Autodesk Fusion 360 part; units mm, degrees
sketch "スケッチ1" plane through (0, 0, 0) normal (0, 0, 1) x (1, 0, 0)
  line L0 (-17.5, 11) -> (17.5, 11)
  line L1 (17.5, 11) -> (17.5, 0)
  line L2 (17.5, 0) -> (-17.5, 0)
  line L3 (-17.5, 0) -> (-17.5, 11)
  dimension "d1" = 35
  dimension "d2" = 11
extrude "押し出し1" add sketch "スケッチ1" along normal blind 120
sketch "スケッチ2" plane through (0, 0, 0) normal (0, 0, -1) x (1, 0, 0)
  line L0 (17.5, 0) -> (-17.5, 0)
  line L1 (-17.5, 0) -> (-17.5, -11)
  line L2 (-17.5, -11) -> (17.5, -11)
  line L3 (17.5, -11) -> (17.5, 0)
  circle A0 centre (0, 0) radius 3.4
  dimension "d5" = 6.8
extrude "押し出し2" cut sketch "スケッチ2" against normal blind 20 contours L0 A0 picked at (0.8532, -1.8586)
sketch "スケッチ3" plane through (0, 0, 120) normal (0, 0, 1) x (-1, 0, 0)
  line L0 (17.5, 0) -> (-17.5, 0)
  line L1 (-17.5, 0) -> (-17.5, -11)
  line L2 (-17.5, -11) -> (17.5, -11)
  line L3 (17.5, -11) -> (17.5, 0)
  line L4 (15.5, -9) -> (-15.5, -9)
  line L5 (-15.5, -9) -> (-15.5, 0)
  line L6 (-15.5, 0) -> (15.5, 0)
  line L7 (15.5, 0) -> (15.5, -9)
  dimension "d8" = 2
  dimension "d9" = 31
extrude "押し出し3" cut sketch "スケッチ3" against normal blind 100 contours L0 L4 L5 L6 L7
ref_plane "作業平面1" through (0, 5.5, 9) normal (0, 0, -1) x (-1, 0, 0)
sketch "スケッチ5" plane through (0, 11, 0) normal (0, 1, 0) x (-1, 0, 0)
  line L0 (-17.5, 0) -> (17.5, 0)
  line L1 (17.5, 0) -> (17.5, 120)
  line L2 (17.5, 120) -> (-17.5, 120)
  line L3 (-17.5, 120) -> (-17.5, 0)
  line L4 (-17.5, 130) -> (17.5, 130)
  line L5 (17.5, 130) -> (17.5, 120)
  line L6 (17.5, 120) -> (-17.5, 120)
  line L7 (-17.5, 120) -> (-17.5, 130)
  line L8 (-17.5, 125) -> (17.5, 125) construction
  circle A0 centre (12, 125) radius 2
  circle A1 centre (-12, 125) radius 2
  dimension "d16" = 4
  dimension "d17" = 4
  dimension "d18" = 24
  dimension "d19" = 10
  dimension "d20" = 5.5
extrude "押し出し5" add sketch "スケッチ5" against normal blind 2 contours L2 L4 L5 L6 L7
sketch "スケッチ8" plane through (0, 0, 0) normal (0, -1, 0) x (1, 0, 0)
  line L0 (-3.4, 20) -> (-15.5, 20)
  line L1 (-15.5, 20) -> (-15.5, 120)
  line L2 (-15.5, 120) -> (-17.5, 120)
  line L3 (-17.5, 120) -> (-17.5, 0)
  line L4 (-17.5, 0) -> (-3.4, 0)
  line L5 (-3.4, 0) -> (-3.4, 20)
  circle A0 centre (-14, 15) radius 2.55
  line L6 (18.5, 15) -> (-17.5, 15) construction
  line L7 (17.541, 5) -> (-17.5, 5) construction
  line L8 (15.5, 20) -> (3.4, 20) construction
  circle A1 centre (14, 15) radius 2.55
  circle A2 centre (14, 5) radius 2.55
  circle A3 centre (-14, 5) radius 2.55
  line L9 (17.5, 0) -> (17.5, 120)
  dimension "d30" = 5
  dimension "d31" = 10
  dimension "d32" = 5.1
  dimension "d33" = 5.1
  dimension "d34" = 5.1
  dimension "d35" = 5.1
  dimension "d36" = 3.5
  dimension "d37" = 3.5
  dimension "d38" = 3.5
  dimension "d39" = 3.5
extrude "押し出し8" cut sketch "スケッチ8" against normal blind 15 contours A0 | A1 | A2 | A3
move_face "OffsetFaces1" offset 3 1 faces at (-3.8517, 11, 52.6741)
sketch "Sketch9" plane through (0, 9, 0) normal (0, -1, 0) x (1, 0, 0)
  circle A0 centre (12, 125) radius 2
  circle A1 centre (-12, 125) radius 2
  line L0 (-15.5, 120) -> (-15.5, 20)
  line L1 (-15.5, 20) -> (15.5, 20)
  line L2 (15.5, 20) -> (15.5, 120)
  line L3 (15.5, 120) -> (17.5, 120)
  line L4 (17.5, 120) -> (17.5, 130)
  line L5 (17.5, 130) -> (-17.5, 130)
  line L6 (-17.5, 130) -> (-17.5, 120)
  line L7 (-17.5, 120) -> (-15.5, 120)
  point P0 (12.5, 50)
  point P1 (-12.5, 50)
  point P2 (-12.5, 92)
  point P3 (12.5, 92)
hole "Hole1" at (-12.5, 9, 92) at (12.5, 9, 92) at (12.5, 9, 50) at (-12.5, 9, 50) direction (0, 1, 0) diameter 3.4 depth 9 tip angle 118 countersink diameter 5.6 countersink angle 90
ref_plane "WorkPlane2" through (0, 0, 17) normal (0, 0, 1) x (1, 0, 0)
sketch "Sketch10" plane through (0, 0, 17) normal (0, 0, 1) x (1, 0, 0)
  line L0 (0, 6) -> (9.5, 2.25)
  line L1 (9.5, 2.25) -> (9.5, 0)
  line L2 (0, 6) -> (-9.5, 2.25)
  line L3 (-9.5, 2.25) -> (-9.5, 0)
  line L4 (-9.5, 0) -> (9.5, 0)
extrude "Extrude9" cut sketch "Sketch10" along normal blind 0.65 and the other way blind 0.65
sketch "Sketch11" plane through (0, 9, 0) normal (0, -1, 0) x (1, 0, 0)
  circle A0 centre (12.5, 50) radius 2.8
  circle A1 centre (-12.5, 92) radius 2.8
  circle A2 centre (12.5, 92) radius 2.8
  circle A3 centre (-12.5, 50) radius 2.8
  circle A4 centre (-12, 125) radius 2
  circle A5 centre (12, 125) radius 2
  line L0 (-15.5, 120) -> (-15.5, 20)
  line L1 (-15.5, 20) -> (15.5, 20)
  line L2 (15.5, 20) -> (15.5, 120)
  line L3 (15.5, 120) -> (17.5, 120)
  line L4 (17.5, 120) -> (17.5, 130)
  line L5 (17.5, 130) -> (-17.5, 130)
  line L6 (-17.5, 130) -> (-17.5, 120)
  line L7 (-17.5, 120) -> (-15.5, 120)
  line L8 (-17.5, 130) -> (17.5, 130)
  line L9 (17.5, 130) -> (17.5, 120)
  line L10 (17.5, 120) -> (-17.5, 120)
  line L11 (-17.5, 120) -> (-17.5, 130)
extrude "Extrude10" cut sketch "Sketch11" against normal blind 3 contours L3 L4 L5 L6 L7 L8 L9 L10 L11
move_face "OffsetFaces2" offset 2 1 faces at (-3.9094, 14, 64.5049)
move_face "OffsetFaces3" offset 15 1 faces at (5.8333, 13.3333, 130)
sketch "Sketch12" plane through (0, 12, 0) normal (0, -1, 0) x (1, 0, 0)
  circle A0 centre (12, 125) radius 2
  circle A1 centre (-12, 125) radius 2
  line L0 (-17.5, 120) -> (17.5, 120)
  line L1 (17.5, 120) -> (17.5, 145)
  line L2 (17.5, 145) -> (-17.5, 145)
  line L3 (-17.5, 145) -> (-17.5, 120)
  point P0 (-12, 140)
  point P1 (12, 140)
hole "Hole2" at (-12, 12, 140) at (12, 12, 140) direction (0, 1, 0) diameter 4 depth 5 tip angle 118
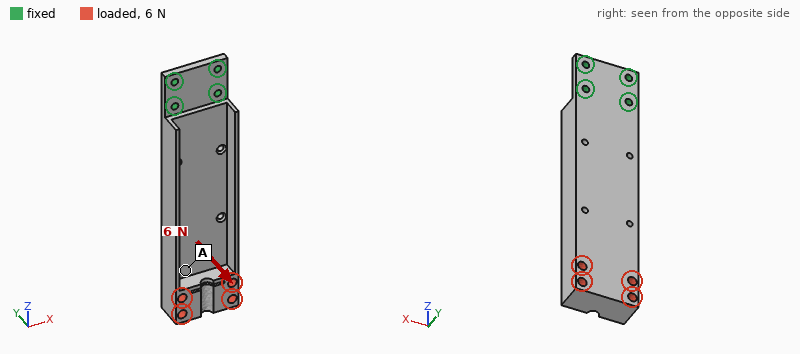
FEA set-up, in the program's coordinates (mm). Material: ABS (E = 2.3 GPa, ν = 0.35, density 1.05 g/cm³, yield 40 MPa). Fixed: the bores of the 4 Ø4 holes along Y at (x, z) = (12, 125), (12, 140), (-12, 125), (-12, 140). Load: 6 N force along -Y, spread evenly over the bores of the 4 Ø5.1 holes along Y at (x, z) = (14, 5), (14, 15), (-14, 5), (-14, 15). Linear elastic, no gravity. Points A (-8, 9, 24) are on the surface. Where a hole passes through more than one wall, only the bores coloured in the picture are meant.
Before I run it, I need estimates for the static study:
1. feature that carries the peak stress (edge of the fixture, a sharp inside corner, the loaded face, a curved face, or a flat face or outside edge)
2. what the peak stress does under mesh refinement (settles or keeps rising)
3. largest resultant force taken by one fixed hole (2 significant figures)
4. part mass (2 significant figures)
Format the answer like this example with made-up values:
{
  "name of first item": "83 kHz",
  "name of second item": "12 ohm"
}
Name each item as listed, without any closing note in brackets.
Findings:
{
  "feature that carries the peak stress": "edge of the fixture",
  "what the peak stress does under mesh refinement": "keeps rising",
  "largest resultant force taken by one fixed hole": "11 N",
  "part mass": "43 g"
}
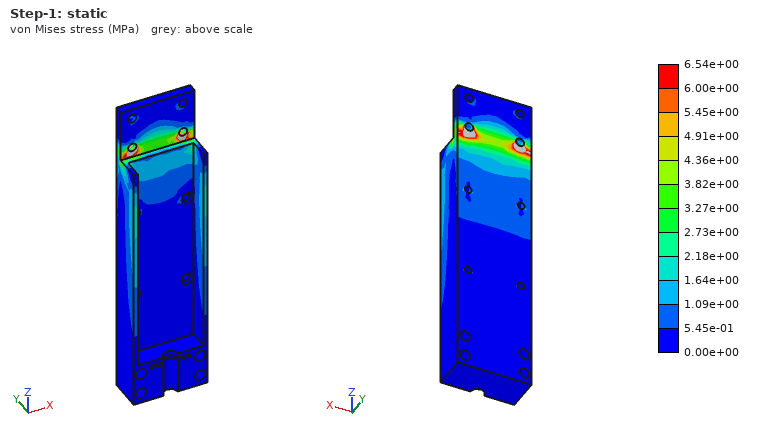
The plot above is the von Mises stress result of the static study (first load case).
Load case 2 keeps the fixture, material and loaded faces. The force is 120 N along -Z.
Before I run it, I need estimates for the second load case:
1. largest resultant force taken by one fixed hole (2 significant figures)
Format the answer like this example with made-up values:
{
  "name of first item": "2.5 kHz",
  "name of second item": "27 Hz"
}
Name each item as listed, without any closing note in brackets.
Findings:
{
  "largest resultant force taken by one fixed hole": "51 N"
}
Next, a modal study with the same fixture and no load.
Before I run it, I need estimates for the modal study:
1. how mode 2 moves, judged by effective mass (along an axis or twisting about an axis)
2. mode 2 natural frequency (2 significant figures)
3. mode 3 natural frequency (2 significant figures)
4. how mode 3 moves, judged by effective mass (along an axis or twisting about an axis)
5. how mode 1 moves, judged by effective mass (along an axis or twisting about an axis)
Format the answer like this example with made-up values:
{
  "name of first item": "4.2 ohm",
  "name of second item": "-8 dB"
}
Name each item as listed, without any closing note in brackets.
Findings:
{
  "how mode 2 moves, judged by effective mass": "along X",
  "mode 2 natural frequency": "380 Hz",
  "mode 3 natural frequency": "530 Hz",
  "how mode 3 moves, judged by effective mass": "twisting about Z",
  "how mode 1 moves, judged by effective mass": "along Y"
}
